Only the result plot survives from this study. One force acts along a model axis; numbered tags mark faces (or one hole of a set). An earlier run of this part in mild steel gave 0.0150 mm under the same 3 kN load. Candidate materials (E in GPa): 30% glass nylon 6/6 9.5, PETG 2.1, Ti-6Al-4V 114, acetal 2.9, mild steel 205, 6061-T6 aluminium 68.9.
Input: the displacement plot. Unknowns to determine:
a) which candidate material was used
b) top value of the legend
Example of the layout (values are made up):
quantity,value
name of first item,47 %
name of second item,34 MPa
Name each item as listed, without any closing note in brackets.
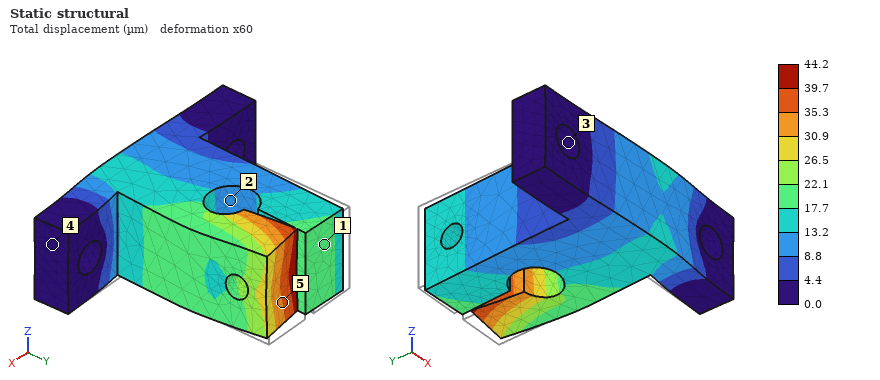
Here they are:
quantity,value
which candidate material was used,6061-T6 aluminium
top value of the legend,44.2 µm
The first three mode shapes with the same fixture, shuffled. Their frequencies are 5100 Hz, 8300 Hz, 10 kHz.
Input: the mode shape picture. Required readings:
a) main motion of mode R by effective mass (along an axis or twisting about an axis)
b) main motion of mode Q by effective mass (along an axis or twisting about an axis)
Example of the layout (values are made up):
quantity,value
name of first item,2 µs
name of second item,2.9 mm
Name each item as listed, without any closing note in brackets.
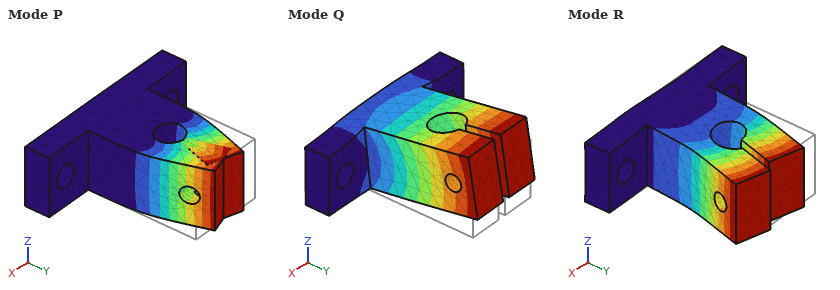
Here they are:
quantity,value
main motion of mode R by effective mass,along X
main motion of mode Q by effective mass,along Z
